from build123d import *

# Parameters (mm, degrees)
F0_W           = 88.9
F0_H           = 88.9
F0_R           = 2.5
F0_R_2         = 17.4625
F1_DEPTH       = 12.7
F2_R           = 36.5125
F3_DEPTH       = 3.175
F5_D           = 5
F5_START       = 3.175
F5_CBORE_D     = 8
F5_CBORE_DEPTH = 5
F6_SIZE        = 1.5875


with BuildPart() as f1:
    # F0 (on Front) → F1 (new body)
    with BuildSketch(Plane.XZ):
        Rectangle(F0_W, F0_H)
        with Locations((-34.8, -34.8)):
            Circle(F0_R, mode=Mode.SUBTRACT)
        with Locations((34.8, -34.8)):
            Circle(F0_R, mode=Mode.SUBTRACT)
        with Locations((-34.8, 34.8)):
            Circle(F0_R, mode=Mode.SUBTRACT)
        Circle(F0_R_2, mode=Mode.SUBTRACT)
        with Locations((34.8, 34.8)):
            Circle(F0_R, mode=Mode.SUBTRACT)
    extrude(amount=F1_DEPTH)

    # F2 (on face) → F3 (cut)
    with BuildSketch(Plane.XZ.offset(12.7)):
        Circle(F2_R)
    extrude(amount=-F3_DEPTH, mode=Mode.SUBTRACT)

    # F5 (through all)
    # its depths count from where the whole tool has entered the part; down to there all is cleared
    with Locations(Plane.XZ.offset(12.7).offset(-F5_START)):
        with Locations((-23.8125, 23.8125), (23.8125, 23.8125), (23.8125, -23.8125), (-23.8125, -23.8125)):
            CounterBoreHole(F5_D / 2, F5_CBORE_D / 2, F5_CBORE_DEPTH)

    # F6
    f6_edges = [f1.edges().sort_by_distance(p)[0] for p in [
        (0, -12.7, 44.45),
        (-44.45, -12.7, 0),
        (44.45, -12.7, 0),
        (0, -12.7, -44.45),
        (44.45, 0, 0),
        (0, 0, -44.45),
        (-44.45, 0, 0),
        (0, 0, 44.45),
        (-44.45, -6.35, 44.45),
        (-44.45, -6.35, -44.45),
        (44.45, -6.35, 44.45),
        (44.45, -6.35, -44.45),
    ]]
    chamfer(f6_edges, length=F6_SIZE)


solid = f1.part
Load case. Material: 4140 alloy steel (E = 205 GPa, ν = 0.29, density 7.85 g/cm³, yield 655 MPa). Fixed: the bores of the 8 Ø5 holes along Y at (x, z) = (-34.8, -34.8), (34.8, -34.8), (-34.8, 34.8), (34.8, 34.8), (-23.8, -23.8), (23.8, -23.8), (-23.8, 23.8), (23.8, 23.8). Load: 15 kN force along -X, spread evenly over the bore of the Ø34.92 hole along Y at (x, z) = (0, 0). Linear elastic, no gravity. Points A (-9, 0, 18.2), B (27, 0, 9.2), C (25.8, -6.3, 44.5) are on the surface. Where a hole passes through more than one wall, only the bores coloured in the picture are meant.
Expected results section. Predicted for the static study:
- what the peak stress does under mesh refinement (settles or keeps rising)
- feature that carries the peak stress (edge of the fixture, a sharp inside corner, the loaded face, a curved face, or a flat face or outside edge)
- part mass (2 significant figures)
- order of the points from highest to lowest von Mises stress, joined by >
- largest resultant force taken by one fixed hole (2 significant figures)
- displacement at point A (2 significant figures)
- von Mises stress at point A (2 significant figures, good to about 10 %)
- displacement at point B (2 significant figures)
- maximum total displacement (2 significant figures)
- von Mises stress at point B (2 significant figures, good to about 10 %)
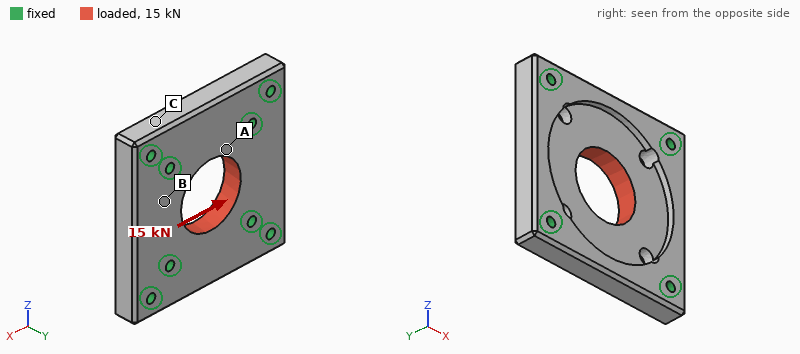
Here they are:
keeps rising
edge of the fixture
590 g
A > B > C
2.5 kN
1.9 µm
23 MPa
2.2 µm
3.5 µm
12 MPa
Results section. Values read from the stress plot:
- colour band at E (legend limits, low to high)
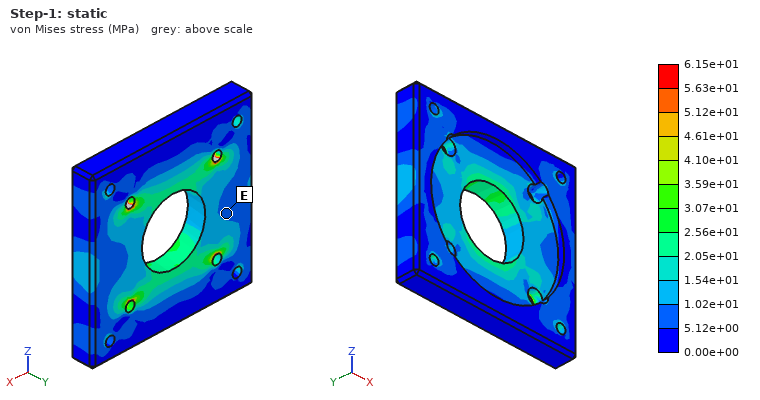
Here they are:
5.12e+00 to 1.02e+01 MPa
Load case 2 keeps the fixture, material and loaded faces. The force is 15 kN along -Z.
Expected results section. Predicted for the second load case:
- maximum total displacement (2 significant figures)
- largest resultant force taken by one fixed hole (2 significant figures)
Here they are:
3.5 µm
2.5 kN
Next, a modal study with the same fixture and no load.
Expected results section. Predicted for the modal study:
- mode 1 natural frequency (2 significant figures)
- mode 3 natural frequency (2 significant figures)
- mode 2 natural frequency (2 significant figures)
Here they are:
12 kHz
14 kHz
14 kHz
